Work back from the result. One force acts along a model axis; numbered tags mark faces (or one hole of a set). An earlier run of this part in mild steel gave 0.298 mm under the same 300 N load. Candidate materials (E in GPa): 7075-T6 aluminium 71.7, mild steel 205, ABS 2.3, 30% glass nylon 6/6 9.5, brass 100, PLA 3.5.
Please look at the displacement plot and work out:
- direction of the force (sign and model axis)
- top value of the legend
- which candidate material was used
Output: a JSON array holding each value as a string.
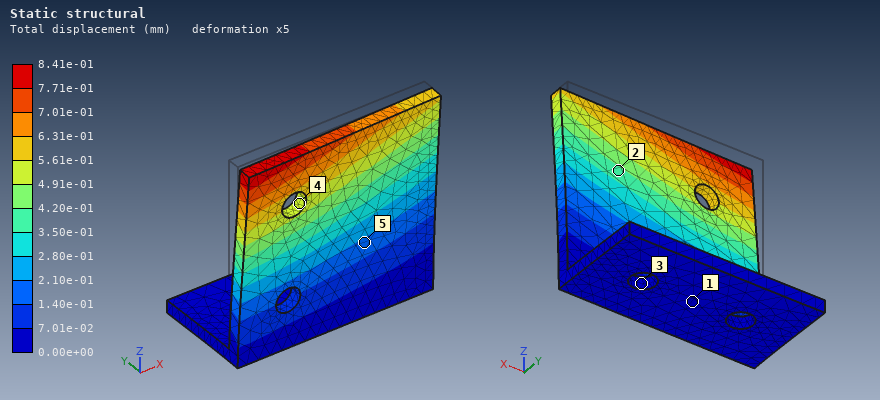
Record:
["-Y", "8.41e-01 mm", "7075-T6 aluminium"]
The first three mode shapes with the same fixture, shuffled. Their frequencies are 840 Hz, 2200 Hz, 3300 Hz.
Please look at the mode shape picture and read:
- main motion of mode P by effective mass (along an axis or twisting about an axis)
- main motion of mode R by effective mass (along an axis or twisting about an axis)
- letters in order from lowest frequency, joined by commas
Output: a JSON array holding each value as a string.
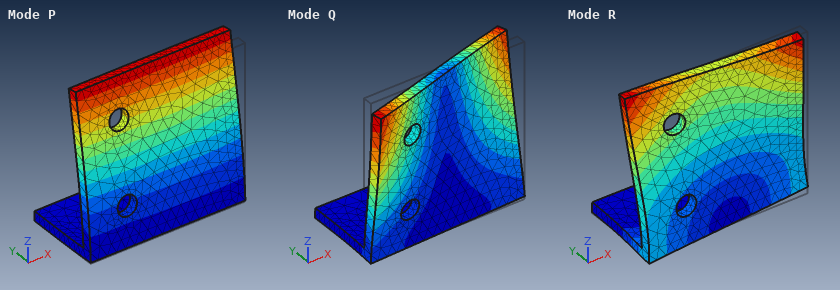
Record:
["along Y", "along X", "P, Q, R"]
